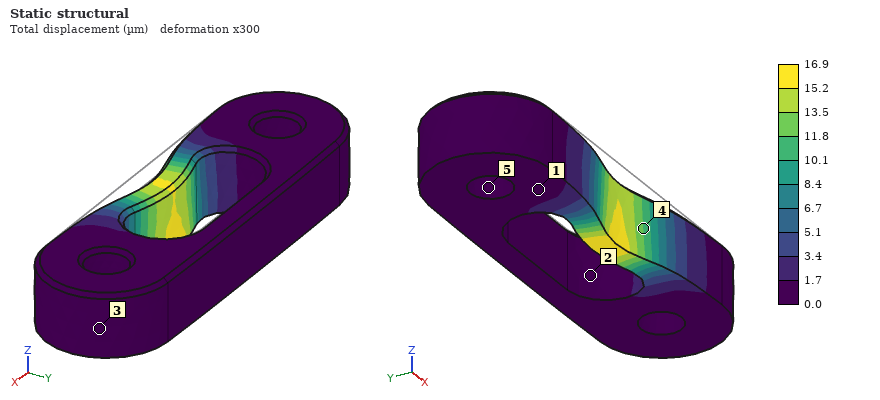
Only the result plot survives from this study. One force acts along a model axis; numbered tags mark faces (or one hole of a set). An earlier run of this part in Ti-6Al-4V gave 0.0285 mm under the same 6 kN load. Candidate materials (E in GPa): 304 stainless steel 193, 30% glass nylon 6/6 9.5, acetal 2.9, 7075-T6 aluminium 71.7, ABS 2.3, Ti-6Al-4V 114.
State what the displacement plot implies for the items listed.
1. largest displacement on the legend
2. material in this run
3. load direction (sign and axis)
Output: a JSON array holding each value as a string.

["16.9 µm", "304 stainless steel", "+Y"]
